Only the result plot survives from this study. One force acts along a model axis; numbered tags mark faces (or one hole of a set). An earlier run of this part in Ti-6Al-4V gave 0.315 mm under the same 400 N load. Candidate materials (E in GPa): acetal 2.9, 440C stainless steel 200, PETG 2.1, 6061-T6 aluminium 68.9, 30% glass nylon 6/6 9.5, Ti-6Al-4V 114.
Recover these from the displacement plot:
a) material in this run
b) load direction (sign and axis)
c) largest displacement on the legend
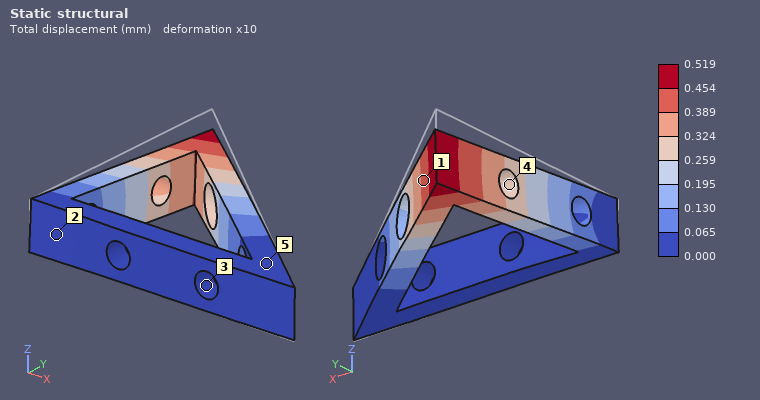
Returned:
6061-T6 aluminium
-Z
0.519 mm
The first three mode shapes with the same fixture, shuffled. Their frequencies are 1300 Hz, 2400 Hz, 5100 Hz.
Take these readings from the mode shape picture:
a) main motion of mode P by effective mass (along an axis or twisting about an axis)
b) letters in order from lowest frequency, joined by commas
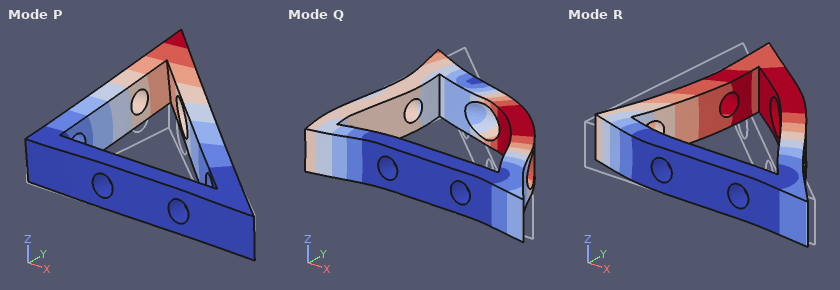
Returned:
along Z
P, R, Q
